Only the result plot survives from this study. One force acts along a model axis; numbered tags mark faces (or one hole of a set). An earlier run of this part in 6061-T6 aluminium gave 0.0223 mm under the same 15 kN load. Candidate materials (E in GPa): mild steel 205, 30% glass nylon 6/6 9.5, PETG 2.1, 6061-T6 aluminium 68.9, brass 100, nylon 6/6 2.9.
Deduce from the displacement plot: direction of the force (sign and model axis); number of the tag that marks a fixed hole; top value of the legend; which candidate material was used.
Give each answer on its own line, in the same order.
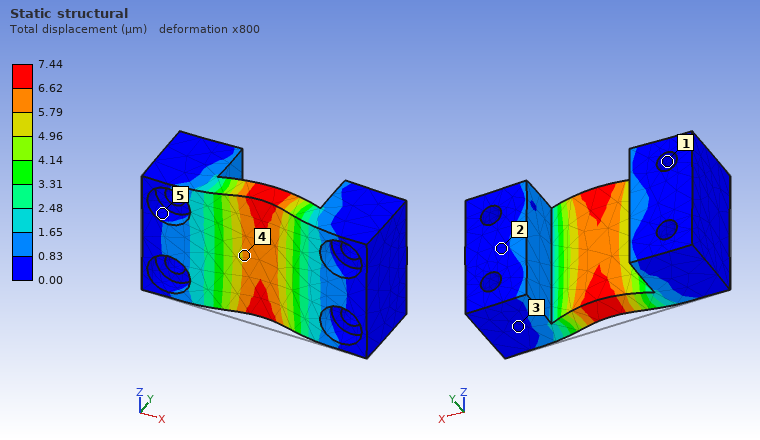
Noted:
+Y
1
7.44 µm
mild steel
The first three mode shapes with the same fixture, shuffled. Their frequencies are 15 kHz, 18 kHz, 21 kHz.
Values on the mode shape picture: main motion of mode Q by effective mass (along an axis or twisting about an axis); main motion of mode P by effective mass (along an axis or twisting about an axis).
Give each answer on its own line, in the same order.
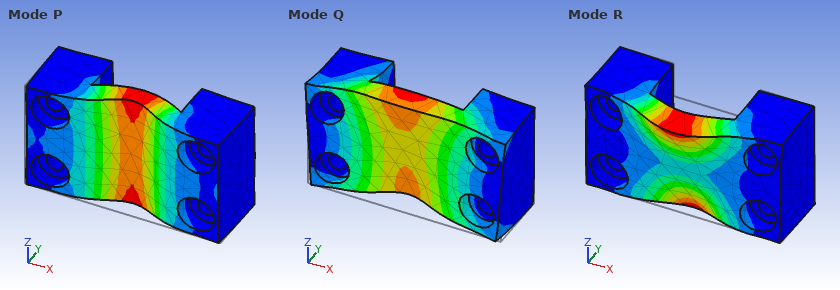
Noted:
along Z
along Y
